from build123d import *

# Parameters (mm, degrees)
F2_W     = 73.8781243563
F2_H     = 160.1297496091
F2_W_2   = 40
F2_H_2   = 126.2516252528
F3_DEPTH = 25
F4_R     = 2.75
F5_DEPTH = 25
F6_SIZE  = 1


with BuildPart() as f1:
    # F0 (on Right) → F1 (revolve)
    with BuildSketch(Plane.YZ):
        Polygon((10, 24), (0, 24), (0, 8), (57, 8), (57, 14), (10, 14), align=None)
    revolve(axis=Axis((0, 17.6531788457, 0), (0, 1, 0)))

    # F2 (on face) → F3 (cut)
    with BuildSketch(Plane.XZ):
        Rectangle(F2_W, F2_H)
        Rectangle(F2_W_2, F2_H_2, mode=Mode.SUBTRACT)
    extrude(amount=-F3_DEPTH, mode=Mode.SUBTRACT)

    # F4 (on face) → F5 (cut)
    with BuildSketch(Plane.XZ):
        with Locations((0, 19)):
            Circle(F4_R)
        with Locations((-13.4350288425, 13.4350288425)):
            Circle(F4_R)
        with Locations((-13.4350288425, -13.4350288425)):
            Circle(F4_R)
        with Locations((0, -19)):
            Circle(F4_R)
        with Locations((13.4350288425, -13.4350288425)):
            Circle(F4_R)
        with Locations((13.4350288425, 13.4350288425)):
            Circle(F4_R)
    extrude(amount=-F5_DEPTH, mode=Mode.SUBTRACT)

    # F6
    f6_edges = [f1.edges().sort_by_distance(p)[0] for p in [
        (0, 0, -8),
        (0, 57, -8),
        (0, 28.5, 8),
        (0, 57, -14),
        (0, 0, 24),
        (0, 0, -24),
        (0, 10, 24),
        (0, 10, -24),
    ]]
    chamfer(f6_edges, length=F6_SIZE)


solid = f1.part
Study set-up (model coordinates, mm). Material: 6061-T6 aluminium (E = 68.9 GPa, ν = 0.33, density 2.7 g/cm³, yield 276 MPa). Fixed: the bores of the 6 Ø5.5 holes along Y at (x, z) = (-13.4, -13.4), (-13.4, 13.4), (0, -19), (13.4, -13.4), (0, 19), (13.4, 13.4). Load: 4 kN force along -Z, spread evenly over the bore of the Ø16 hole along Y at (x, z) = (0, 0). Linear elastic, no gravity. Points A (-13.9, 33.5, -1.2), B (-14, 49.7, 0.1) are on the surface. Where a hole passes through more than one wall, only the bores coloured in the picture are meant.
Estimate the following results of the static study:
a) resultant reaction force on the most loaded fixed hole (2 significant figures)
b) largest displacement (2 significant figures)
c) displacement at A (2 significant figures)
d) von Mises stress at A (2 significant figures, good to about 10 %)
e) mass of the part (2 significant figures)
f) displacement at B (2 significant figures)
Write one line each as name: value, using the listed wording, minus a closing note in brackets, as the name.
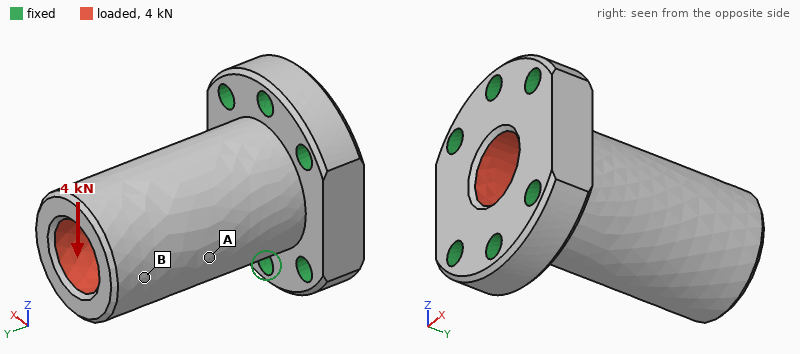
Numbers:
resultant reaction force on the most loaded fixed hole: 1.7 kN
largest displacement: 48 µm
displacement at A: 23 µm
von Mises stress at A: 11 MPa
mass of the part: 88 g
displacement at B: 40 µm
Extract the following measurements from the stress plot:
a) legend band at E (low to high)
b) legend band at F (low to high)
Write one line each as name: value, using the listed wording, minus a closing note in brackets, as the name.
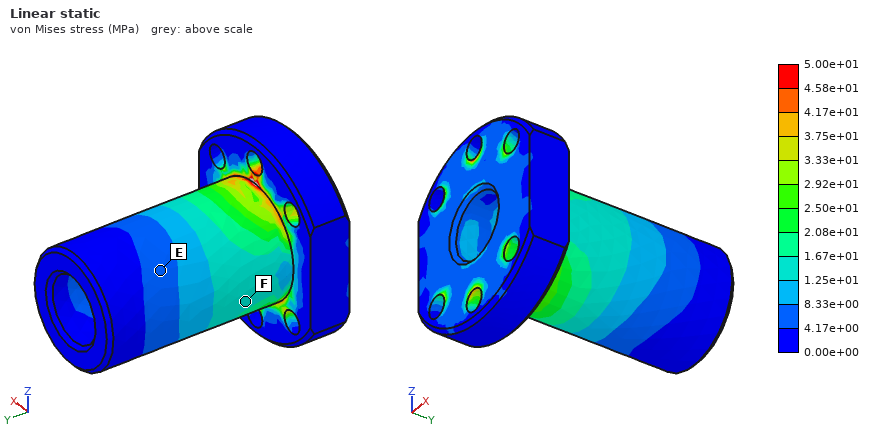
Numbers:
legend band at E: 4.17e+00 to 8.33e+00 MPa
legend band at F: 1.25e+01 to 1.67e+01 MPa
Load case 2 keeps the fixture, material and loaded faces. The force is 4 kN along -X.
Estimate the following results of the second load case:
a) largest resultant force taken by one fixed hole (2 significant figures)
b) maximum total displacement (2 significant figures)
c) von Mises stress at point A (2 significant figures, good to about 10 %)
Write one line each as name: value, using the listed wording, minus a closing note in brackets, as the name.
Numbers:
largest resultant force taken by one fixed hole: 2.0 kN
maximum total displacement: 56 µm
von Mises stress at point A: 9.4 MPa
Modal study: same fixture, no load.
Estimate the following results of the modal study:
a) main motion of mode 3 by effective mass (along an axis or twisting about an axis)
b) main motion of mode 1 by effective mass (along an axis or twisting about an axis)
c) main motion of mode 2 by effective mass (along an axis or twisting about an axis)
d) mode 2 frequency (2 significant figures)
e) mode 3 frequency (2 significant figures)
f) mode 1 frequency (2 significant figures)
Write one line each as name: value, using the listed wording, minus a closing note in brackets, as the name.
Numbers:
main motion of mode 3 by effective mass: twisting about Y
main motion of mode 1 by effective mass: along X
main motion of mode 2 by effective mass: along Z
mode 2 frequency: 6800 Hz
mode 3 frequency: 15 kHz
mode 1 frequency: 6400 Hz
